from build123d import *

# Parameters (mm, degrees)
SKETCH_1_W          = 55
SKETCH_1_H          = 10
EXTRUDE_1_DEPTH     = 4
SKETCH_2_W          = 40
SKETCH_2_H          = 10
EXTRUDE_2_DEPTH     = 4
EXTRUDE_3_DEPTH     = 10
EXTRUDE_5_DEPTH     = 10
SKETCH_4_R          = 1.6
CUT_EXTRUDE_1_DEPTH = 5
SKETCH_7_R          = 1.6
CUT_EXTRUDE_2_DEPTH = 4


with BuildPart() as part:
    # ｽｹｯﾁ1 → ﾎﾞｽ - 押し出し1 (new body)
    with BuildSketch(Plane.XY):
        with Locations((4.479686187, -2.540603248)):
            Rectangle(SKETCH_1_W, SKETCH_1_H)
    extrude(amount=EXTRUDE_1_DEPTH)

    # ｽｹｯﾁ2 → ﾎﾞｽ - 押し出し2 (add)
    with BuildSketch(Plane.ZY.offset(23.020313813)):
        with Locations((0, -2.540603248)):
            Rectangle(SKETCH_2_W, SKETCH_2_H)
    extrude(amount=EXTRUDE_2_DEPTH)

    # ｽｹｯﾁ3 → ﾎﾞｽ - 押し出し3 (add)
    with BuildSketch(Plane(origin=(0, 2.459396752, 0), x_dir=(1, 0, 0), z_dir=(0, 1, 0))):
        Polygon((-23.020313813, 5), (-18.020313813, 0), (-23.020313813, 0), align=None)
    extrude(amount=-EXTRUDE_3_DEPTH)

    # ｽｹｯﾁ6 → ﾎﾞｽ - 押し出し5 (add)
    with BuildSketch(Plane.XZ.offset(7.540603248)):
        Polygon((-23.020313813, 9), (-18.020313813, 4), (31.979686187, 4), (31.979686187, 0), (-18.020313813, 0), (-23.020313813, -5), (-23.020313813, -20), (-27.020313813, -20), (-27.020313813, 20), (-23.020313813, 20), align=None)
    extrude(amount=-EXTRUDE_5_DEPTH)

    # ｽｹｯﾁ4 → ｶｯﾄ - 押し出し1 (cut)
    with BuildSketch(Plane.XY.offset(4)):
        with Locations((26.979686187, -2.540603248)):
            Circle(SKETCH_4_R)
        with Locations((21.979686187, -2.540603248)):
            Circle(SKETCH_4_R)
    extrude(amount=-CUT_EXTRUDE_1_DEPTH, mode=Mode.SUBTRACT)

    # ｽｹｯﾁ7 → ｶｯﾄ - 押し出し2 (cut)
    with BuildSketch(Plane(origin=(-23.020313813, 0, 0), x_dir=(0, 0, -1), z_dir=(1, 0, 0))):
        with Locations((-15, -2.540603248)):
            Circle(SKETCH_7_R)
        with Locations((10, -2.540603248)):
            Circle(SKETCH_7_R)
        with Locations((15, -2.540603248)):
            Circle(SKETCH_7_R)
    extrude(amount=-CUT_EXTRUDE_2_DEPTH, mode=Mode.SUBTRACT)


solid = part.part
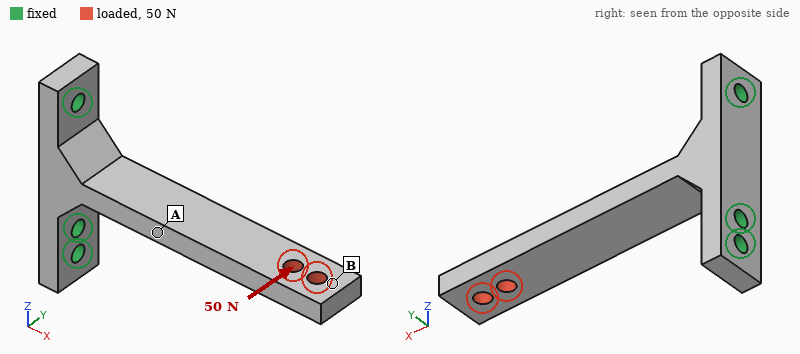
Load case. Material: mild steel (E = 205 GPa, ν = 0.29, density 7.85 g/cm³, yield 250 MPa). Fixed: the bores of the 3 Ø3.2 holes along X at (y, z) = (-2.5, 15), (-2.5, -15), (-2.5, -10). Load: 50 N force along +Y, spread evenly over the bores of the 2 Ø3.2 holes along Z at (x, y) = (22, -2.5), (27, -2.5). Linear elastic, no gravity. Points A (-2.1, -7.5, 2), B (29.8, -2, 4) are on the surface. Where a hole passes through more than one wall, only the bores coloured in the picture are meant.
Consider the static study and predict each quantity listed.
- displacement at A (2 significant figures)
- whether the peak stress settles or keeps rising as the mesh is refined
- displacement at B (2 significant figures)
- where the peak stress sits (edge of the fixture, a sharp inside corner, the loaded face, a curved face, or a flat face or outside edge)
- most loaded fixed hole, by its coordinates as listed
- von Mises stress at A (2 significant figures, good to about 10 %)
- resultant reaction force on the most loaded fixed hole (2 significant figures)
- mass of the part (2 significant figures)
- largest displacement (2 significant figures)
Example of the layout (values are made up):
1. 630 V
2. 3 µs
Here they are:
1. 20 µm
2. keeps rising
3. 60 µm
4. edge of the fixture
5. (-2.5, -10)
6. 20 MPa
7. 62 N
8. 31 g
9. 63 µm
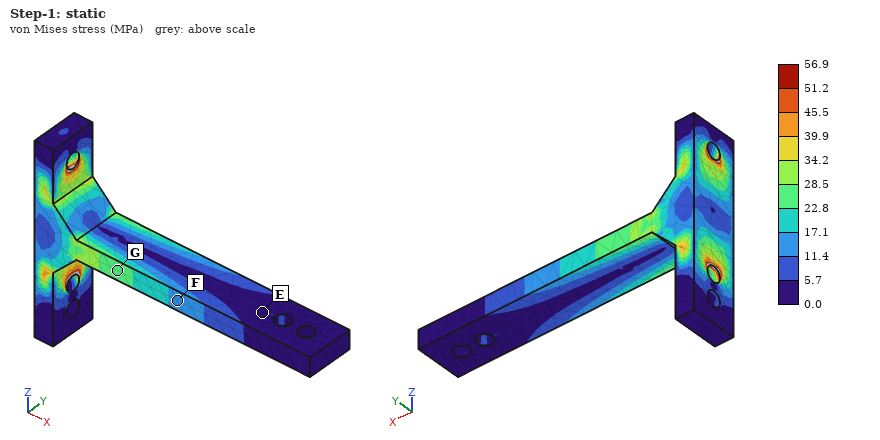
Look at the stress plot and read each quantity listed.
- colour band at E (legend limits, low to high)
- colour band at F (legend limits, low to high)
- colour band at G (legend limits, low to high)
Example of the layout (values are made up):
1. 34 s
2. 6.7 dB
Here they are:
1. 0.0 to 5.7 MPa
2. 11.4 to 17.1 MPa
3. 22.8 to 28.5 MPa
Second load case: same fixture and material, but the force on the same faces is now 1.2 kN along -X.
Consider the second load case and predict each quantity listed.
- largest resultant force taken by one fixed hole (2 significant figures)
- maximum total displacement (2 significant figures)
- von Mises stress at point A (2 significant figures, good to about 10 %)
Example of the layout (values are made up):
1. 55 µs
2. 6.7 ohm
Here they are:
1. 730 N
2. 12 µm
3. 30 MPa
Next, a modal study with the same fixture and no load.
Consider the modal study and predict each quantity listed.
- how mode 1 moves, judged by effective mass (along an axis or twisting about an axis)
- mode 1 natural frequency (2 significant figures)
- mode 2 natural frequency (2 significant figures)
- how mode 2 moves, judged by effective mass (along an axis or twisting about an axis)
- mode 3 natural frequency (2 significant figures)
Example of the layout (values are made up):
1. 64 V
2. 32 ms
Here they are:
1. along Z
2. 1300 Hz
3. 1900 Hz
4. along Y
5. 7400 Hz
